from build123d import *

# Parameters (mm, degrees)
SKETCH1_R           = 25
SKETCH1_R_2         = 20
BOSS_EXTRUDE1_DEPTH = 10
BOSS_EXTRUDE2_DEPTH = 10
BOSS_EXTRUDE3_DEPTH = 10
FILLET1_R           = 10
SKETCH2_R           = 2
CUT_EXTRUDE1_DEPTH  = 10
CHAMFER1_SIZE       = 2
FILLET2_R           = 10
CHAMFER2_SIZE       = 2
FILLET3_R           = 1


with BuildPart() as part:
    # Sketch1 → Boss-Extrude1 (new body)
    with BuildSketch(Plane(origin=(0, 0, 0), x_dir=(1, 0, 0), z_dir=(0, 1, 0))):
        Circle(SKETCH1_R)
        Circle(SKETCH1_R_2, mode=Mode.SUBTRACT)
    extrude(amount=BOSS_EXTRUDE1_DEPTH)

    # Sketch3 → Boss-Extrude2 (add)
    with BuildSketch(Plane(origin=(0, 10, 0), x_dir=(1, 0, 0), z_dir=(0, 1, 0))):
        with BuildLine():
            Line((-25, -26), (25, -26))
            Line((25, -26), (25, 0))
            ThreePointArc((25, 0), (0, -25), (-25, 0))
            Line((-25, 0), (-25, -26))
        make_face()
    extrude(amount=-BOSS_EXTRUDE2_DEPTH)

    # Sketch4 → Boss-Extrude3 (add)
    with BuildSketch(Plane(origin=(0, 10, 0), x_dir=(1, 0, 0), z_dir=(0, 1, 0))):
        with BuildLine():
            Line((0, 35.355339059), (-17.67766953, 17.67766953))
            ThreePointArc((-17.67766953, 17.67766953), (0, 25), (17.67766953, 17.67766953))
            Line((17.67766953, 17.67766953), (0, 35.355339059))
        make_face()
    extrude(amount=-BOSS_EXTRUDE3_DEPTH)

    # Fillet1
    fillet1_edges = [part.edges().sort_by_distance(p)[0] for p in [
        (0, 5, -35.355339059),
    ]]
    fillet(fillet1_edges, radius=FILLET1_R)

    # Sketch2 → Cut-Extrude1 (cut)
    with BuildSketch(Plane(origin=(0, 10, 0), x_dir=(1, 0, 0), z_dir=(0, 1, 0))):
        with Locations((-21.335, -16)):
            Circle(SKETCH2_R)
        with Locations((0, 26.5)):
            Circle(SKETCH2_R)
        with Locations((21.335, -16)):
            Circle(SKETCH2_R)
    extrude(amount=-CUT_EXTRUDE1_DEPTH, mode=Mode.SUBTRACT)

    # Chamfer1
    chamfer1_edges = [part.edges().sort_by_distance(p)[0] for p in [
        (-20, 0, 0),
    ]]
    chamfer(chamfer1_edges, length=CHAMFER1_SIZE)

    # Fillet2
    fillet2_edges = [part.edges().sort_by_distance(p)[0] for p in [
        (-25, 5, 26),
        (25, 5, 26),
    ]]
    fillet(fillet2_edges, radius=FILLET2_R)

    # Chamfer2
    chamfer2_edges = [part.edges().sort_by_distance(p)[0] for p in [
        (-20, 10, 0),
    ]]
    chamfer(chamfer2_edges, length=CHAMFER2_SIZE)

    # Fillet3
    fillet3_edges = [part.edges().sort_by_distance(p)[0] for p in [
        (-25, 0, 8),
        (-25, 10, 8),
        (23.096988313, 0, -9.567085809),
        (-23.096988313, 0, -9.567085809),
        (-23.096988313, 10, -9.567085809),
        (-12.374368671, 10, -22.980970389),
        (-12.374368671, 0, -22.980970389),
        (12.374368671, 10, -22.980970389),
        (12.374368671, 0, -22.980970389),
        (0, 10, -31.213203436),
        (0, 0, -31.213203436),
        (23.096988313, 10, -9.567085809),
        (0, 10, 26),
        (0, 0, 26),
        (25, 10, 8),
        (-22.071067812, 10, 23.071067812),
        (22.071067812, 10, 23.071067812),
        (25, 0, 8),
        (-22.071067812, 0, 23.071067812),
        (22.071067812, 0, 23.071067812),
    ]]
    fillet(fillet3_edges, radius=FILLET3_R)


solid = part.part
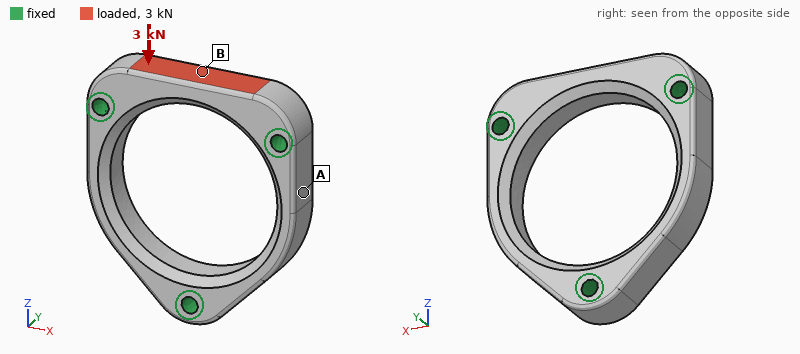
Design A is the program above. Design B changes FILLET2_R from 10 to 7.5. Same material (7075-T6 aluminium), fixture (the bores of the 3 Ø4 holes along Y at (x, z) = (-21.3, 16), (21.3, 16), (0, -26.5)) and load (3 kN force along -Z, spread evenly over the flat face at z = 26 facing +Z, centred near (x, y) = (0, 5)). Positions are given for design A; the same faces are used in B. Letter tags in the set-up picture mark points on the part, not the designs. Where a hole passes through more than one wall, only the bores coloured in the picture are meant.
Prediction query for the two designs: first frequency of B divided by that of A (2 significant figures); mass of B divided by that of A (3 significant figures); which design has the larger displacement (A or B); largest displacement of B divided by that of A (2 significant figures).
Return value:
1.00
1.02
A
0.88
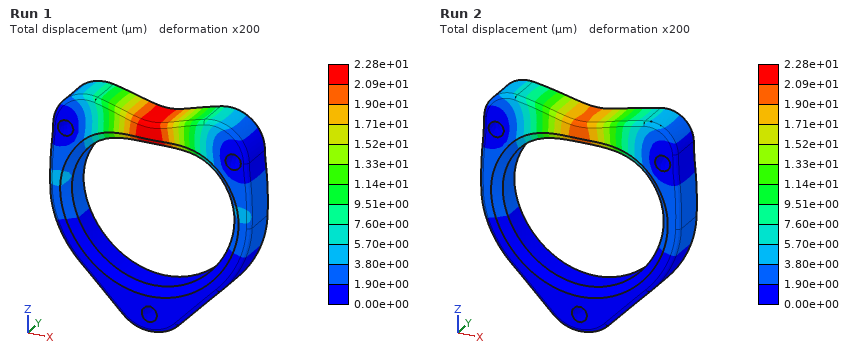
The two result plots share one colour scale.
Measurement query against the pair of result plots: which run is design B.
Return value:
Run 2
